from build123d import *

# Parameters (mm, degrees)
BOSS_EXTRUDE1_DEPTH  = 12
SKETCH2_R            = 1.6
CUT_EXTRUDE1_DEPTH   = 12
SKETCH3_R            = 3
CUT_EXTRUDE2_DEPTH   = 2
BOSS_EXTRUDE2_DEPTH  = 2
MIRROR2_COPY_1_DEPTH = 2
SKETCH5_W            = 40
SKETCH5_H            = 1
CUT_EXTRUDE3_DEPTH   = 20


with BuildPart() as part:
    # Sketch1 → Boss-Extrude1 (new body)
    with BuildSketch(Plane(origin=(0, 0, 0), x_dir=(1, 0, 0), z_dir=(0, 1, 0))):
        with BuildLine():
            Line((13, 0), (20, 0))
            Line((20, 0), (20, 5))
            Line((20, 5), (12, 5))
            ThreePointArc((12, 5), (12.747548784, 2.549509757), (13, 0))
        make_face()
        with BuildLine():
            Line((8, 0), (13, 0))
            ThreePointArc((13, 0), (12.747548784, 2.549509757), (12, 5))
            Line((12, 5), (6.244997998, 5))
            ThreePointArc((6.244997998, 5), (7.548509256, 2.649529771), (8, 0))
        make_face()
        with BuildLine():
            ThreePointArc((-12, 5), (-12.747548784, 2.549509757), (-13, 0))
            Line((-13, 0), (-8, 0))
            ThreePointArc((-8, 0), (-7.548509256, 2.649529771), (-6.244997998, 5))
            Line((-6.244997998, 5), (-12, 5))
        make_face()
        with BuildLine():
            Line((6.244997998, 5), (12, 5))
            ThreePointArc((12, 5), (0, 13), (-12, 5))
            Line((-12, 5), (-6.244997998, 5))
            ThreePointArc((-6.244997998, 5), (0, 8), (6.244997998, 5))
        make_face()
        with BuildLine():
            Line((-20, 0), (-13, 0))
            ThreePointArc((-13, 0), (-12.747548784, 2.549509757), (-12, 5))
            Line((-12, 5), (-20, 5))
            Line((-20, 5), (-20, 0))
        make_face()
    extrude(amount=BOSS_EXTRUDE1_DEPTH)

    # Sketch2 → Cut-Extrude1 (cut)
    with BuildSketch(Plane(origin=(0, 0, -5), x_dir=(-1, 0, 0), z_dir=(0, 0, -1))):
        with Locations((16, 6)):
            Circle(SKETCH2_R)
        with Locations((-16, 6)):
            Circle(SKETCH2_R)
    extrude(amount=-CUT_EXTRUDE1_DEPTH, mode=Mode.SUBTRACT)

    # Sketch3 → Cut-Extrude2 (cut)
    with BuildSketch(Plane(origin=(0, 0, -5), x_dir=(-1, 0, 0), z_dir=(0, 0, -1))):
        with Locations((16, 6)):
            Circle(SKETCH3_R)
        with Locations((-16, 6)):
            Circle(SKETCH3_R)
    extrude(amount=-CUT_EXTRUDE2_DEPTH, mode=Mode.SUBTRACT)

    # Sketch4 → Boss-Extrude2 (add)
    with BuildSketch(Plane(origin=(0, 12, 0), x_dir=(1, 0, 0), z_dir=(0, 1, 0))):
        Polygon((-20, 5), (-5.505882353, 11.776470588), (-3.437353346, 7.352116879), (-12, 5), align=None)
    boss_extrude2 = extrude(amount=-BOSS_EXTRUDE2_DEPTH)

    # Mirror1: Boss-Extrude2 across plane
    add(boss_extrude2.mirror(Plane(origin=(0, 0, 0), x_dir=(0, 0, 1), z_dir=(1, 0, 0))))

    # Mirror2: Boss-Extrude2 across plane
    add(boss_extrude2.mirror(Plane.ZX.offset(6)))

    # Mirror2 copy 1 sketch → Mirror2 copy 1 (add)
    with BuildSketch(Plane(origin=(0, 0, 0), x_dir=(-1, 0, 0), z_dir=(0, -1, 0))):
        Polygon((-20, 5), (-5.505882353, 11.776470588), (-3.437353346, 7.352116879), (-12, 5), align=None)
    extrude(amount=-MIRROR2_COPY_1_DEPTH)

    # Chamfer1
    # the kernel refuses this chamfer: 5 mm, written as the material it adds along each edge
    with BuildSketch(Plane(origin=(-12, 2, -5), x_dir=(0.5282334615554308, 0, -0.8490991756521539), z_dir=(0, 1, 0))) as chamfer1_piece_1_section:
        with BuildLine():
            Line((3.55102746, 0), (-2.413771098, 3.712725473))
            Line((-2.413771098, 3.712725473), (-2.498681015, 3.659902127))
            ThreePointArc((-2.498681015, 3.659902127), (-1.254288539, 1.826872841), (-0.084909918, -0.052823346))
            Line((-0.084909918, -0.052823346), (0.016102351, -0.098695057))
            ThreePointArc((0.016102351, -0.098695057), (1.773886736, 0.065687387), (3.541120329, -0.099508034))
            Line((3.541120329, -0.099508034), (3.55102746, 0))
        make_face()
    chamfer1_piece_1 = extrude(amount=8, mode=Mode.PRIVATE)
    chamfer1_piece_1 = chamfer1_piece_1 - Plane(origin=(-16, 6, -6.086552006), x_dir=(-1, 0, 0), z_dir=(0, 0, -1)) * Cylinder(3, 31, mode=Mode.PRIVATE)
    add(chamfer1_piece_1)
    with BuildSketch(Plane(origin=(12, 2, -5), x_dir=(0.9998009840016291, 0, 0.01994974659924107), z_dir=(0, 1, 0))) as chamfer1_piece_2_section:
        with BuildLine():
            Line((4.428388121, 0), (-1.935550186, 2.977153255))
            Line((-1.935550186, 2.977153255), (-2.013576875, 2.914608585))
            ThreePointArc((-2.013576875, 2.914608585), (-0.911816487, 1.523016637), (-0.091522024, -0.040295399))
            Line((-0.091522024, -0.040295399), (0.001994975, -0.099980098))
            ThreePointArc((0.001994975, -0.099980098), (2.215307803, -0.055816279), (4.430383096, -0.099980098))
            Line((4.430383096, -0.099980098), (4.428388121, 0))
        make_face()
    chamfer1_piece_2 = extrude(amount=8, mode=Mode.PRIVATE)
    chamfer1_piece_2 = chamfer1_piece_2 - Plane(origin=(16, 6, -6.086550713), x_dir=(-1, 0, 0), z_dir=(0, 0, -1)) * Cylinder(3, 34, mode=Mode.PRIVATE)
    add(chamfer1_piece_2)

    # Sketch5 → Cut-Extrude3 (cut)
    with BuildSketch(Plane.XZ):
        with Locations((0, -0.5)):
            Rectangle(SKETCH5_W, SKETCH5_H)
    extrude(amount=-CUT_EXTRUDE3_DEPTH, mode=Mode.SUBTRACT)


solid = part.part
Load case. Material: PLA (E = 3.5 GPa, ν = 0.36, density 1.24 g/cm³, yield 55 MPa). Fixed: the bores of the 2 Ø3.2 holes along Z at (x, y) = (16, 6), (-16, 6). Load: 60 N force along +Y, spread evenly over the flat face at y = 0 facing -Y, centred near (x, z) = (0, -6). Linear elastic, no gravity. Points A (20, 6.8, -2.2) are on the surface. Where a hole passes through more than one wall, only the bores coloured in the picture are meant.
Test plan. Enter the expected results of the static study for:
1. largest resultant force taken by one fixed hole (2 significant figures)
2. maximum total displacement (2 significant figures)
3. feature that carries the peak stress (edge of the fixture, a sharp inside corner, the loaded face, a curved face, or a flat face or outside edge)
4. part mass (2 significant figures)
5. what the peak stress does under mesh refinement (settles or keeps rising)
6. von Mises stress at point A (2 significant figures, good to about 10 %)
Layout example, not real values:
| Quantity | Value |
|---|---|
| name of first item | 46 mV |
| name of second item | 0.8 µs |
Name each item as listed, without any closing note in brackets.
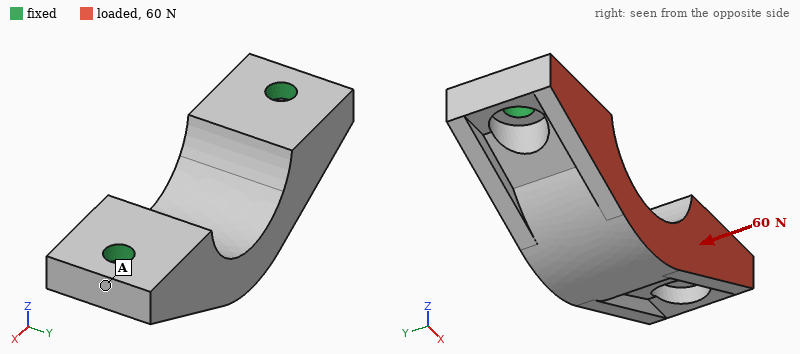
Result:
| Quantity | Value |
|---|---|
| largest resultant force taken by one fixed hole | 30 N |
| maximum total displacement | 62 µm |
| feature that carries the peak stress | edge of the fixture |
| part mass | 3.3 g |
| what the peak stress does under mesh refinement | keeps rising |
| von Mises stress at point A | 2.0 MPa |
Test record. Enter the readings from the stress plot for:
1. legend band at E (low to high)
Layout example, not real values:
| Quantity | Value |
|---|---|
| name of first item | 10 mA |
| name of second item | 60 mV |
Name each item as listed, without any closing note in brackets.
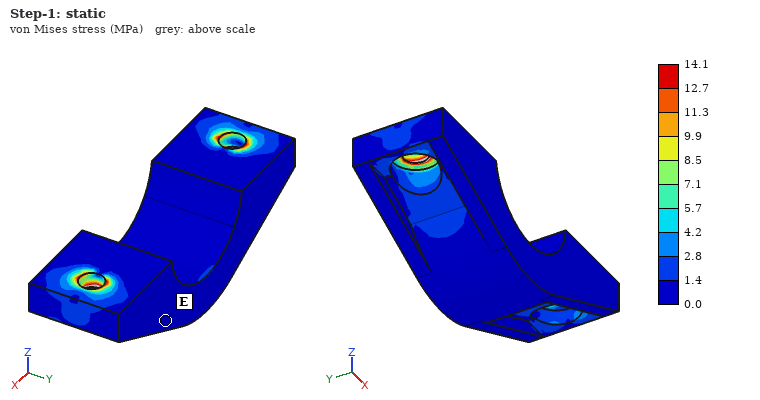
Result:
| Quantity | Value |
|---|---|
| legend band at E | 0.0 to 1.4 MPa |
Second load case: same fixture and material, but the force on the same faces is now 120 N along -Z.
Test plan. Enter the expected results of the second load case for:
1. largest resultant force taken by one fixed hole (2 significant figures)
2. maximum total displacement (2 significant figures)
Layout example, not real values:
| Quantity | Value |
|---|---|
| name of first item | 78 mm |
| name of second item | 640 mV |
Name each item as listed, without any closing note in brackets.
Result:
| Quantity | Value |
|---|---|
| largest resultant force taken by one fixed hole | 70 N |
| maximum total displacement | 0.14 mm |
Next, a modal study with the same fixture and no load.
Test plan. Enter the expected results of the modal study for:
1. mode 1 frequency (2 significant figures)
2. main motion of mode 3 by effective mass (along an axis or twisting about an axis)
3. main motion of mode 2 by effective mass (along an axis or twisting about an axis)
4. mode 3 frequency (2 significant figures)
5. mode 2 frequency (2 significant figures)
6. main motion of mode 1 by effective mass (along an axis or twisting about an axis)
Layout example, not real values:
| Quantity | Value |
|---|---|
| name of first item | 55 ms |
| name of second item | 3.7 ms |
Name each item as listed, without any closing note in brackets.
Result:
| Quantity | Value |
|---|---|
| mode 1 frequency | 3200 Hz |
| main motion of mode 3 by effective mass | along X |
| main motion of mode 2 by effective mass | along Z |
| mode 3 frequency | 10 kHz |
| mode 2 frequency | 8300 Hz |
| main motion of mode 1 by effective mass | along Y |
